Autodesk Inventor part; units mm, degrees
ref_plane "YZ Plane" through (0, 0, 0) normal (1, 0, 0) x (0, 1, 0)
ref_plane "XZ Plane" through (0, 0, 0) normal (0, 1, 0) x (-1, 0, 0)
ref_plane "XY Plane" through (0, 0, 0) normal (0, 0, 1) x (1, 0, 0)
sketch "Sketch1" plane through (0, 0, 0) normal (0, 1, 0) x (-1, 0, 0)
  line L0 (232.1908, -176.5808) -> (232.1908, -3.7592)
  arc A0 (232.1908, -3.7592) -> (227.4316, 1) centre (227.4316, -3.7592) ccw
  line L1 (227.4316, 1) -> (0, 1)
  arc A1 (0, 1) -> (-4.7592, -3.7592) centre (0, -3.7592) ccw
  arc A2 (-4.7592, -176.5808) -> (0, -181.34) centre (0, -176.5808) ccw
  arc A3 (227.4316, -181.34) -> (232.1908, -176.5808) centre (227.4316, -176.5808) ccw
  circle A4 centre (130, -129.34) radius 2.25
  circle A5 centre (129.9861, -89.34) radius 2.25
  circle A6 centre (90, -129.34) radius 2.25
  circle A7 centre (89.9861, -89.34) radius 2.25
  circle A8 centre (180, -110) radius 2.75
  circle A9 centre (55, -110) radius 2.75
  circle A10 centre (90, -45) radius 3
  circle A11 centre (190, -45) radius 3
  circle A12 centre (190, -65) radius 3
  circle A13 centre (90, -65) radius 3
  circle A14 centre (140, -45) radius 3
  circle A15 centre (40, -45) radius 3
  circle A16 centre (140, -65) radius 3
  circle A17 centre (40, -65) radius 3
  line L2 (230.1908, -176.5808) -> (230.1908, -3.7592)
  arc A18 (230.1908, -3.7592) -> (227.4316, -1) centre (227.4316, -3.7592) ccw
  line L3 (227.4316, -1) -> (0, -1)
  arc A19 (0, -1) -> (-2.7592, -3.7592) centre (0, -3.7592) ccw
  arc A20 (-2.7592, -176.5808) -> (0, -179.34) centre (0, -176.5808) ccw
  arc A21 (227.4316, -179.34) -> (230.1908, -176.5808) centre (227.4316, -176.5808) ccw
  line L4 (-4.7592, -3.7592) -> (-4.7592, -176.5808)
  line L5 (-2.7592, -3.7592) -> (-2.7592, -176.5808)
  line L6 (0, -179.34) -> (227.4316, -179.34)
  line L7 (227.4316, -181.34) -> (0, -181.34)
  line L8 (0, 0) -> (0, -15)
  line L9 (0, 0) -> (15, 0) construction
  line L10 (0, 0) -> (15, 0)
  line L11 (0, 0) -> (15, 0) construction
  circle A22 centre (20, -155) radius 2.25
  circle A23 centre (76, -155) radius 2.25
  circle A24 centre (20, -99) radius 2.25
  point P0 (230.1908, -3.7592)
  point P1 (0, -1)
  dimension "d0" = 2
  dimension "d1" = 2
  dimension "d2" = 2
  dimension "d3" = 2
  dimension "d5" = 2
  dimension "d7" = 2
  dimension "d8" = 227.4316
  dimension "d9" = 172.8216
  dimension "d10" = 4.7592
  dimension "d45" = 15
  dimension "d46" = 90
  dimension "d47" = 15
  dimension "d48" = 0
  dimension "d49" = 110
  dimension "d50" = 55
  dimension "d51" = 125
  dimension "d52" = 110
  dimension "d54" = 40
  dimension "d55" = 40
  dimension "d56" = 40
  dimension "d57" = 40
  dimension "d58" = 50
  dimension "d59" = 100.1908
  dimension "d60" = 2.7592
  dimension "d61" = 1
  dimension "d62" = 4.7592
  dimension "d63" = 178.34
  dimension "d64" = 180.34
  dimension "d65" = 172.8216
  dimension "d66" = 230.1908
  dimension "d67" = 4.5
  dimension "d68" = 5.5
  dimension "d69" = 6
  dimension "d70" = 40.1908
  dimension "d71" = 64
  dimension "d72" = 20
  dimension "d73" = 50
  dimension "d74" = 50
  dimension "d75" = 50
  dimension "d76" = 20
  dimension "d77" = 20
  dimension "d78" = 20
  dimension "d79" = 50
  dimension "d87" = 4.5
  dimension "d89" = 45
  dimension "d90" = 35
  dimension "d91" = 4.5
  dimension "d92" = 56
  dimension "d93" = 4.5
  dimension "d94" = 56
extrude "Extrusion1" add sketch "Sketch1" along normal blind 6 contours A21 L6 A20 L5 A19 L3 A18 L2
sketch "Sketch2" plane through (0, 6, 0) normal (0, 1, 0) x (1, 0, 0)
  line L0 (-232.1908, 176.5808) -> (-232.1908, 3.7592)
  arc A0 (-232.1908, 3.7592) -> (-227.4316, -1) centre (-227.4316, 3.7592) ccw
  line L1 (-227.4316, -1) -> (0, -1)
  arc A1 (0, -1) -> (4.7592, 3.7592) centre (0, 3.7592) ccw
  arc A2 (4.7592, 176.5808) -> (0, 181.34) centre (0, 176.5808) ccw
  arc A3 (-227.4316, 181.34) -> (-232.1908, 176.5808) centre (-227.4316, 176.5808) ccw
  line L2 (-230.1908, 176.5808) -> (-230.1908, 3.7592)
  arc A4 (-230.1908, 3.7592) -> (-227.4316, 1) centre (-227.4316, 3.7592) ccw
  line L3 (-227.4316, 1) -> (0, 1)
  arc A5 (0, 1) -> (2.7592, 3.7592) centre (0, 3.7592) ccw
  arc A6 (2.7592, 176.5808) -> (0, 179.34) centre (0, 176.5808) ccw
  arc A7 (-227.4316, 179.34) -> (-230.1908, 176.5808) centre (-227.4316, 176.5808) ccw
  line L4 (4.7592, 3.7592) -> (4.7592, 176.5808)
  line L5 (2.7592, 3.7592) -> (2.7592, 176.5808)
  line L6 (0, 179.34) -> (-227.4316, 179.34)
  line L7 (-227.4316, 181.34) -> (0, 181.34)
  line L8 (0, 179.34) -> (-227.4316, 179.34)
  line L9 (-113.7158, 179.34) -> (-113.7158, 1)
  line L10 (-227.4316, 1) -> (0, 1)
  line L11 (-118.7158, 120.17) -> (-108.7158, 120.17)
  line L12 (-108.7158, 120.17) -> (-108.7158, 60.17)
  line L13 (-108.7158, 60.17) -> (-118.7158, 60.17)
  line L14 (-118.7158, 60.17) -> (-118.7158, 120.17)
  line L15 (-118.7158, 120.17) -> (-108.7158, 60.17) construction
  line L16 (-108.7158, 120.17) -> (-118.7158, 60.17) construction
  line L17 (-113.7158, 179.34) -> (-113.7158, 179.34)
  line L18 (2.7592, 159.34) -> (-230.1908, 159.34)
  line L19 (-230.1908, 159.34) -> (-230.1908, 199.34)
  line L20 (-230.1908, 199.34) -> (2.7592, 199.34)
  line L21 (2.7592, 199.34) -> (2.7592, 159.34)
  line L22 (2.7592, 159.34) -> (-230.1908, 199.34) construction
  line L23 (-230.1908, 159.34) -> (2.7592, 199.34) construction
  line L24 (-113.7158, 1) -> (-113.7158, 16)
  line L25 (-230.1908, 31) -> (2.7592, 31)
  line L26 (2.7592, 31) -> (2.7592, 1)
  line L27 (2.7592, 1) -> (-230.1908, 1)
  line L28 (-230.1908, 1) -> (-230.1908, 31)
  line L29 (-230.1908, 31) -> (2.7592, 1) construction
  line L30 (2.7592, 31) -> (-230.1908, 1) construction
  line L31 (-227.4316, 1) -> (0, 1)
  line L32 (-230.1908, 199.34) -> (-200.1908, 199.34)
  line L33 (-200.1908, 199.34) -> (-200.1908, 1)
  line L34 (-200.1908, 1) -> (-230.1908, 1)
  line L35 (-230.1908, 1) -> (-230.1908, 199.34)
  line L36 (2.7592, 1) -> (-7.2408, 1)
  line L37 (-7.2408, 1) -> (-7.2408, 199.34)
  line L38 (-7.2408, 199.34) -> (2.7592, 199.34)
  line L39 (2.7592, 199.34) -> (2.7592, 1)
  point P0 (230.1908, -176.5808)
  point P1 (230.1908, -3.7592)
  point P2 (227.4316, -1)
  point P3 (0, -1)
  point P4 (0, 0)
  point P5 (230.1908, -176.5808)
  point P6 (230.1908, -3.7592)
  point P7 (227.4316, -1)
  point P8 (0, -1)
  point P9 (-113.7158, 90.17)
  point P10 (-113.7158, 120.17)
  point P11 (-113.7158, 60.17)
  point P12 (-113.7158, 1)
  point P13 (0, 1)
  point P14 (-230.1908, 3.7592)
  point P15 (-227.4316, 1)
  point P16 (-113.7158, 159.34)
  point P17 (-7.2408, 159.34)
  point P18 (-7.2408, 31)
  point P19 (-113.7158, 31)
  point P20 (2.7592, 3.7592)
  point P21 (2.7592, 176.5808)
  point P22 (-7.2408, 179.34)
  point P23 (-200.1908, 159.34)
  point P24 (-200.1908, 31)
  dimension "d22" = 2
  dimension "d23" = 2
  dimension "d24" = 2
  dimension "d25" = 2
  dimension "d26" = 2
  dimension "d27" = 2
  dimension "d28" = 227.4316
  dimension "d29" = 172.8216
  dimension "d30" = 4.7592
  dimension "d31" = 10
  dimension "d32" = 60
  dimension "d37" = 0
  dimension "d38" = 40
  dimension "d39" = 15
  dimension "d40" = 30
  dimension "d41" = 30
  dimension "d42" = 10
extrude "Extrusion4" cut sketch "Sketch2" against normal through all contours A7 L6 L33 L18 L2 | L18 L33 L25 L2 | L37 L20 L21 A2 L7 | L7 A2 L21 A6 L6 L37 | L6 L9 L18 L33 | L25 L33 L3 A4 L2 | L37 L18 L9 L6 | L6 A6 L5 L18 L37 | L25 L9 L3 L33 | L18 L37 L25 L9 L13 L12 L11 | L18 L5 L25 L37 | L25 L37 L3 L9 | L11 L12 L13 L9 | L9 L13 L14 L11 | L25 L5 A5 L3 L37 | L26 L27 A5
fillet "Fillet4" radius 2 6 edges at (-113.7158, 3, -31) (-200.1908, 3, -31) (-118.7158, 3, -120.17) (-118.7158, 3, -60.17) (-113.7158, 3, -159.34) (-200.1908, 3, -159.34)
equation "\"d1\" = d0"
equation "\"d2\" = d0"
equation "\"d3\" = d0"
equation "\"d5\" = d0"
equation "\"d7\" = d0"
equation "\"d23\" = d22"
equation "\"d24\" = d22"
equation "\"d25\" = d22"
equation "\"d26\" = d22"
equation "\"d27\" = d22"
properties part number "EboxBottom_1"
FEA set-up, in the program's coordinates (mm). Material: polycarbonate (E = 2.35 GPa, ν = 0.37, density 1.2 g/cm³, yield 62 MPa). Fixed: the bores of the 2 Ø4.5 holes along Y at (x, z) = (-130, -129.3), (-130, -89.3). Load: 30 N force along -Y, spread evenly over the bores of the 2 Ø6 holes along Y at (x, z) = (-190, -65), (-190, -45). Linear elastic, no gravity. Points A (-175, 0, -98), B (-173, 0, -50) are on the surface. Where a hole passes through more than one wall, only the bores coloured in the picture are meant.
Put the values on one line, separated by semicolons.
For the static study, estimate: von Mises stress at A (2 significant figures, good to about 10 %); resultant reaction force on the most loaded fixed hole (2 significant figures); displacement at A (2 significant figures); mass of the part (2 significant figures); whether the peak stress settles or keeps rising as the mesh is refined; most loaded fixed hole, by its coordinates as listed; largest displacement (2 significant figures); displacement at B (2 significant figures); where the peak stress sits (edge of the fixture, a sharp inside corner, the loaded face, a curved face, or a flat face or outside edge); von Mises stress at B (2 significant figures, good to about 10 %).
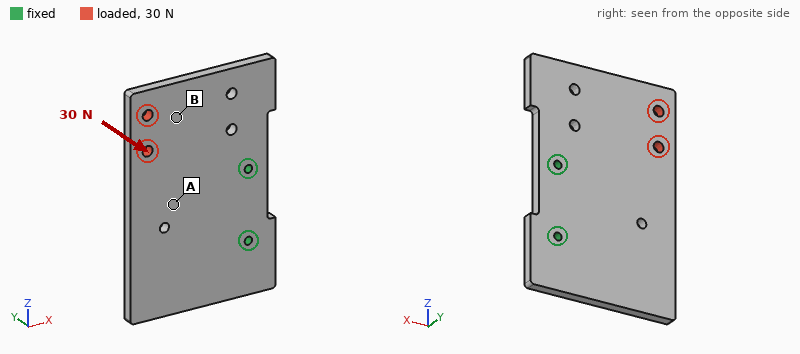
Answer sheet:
2.0 MPa; 44 N; 0.42 mm; 77 g; keeps rising; (-130, -89.3); 1.7 mm; 0.91 mm; edge of the fixture; 1.0 MPa
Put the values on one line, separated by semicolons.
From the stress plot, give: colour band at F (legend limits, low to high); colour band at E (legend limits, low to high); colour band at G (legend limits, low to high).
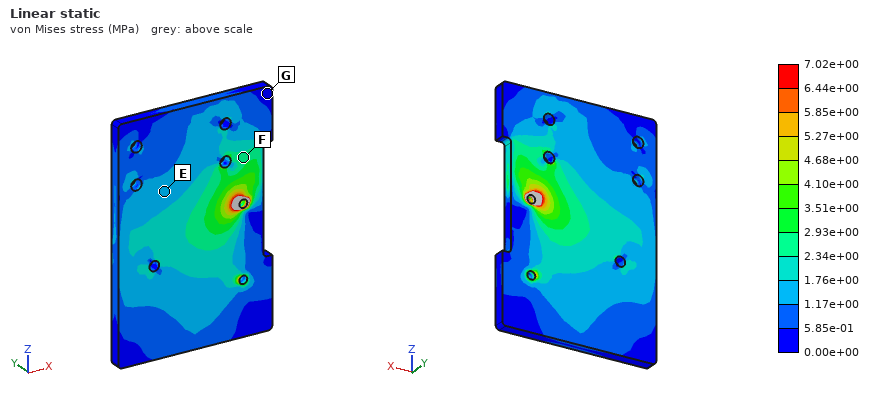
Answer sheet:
2.34e+00 to 2.93e+00 MPa; 1.17e+00 to 1.76e+00 MPa; 0.00e+00 to 5.85e-01 MPa
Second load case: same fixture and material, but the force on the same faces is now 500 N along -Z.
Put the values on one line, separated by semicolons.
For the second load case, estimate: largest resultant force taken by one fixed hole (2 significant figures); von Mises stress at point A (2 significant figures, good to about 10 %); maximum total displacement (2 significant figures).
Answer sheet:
760 N; 2.8 MPa; 0.47 mm
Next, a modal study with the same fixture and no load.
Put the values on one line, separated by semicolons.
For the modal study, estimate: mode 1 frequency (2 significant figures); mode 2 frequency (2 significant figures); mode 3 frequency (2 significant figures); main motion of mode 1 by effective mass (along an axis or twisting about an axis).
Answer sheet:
210 Hz; 290 Hz; 500 Hz; along Y
